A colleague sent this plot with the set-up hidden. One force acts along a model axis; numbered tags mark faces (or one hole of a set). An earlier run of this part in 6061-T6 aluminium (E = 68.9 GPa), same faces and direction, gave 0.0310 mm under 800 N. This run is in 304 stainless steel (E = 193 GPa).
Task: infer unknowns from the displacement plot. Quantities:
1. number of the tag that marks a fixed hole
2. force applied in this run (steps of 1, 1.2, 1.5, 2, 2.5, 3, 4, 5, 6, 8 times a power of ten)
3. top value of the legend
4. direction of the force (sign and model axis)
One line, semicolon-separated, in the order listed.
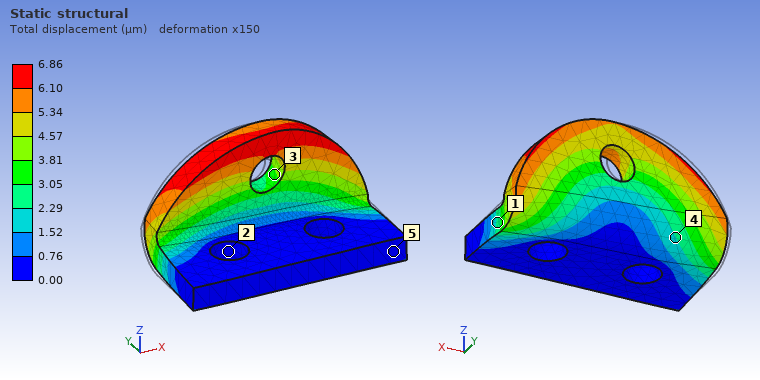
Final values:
2; 500 N; 6.86 µm; +X
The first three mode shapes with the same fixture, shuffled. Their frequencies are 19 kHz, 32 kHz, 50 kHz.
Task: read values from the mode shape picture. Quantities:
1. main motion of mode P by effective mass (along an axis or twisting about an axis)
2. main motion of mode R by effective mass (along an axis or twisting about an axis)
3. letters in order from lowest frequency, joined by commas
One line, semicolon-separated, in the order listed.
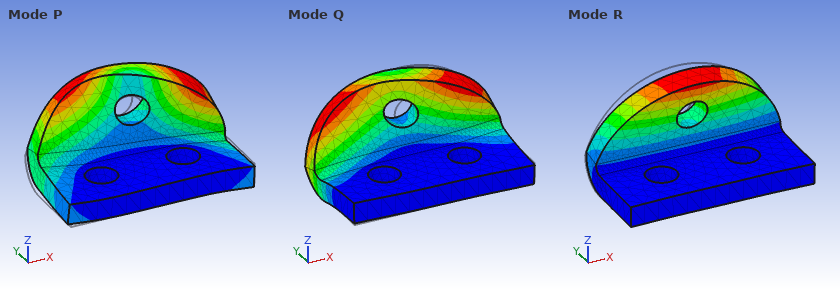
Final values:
along X; along Y; R, Q, P
